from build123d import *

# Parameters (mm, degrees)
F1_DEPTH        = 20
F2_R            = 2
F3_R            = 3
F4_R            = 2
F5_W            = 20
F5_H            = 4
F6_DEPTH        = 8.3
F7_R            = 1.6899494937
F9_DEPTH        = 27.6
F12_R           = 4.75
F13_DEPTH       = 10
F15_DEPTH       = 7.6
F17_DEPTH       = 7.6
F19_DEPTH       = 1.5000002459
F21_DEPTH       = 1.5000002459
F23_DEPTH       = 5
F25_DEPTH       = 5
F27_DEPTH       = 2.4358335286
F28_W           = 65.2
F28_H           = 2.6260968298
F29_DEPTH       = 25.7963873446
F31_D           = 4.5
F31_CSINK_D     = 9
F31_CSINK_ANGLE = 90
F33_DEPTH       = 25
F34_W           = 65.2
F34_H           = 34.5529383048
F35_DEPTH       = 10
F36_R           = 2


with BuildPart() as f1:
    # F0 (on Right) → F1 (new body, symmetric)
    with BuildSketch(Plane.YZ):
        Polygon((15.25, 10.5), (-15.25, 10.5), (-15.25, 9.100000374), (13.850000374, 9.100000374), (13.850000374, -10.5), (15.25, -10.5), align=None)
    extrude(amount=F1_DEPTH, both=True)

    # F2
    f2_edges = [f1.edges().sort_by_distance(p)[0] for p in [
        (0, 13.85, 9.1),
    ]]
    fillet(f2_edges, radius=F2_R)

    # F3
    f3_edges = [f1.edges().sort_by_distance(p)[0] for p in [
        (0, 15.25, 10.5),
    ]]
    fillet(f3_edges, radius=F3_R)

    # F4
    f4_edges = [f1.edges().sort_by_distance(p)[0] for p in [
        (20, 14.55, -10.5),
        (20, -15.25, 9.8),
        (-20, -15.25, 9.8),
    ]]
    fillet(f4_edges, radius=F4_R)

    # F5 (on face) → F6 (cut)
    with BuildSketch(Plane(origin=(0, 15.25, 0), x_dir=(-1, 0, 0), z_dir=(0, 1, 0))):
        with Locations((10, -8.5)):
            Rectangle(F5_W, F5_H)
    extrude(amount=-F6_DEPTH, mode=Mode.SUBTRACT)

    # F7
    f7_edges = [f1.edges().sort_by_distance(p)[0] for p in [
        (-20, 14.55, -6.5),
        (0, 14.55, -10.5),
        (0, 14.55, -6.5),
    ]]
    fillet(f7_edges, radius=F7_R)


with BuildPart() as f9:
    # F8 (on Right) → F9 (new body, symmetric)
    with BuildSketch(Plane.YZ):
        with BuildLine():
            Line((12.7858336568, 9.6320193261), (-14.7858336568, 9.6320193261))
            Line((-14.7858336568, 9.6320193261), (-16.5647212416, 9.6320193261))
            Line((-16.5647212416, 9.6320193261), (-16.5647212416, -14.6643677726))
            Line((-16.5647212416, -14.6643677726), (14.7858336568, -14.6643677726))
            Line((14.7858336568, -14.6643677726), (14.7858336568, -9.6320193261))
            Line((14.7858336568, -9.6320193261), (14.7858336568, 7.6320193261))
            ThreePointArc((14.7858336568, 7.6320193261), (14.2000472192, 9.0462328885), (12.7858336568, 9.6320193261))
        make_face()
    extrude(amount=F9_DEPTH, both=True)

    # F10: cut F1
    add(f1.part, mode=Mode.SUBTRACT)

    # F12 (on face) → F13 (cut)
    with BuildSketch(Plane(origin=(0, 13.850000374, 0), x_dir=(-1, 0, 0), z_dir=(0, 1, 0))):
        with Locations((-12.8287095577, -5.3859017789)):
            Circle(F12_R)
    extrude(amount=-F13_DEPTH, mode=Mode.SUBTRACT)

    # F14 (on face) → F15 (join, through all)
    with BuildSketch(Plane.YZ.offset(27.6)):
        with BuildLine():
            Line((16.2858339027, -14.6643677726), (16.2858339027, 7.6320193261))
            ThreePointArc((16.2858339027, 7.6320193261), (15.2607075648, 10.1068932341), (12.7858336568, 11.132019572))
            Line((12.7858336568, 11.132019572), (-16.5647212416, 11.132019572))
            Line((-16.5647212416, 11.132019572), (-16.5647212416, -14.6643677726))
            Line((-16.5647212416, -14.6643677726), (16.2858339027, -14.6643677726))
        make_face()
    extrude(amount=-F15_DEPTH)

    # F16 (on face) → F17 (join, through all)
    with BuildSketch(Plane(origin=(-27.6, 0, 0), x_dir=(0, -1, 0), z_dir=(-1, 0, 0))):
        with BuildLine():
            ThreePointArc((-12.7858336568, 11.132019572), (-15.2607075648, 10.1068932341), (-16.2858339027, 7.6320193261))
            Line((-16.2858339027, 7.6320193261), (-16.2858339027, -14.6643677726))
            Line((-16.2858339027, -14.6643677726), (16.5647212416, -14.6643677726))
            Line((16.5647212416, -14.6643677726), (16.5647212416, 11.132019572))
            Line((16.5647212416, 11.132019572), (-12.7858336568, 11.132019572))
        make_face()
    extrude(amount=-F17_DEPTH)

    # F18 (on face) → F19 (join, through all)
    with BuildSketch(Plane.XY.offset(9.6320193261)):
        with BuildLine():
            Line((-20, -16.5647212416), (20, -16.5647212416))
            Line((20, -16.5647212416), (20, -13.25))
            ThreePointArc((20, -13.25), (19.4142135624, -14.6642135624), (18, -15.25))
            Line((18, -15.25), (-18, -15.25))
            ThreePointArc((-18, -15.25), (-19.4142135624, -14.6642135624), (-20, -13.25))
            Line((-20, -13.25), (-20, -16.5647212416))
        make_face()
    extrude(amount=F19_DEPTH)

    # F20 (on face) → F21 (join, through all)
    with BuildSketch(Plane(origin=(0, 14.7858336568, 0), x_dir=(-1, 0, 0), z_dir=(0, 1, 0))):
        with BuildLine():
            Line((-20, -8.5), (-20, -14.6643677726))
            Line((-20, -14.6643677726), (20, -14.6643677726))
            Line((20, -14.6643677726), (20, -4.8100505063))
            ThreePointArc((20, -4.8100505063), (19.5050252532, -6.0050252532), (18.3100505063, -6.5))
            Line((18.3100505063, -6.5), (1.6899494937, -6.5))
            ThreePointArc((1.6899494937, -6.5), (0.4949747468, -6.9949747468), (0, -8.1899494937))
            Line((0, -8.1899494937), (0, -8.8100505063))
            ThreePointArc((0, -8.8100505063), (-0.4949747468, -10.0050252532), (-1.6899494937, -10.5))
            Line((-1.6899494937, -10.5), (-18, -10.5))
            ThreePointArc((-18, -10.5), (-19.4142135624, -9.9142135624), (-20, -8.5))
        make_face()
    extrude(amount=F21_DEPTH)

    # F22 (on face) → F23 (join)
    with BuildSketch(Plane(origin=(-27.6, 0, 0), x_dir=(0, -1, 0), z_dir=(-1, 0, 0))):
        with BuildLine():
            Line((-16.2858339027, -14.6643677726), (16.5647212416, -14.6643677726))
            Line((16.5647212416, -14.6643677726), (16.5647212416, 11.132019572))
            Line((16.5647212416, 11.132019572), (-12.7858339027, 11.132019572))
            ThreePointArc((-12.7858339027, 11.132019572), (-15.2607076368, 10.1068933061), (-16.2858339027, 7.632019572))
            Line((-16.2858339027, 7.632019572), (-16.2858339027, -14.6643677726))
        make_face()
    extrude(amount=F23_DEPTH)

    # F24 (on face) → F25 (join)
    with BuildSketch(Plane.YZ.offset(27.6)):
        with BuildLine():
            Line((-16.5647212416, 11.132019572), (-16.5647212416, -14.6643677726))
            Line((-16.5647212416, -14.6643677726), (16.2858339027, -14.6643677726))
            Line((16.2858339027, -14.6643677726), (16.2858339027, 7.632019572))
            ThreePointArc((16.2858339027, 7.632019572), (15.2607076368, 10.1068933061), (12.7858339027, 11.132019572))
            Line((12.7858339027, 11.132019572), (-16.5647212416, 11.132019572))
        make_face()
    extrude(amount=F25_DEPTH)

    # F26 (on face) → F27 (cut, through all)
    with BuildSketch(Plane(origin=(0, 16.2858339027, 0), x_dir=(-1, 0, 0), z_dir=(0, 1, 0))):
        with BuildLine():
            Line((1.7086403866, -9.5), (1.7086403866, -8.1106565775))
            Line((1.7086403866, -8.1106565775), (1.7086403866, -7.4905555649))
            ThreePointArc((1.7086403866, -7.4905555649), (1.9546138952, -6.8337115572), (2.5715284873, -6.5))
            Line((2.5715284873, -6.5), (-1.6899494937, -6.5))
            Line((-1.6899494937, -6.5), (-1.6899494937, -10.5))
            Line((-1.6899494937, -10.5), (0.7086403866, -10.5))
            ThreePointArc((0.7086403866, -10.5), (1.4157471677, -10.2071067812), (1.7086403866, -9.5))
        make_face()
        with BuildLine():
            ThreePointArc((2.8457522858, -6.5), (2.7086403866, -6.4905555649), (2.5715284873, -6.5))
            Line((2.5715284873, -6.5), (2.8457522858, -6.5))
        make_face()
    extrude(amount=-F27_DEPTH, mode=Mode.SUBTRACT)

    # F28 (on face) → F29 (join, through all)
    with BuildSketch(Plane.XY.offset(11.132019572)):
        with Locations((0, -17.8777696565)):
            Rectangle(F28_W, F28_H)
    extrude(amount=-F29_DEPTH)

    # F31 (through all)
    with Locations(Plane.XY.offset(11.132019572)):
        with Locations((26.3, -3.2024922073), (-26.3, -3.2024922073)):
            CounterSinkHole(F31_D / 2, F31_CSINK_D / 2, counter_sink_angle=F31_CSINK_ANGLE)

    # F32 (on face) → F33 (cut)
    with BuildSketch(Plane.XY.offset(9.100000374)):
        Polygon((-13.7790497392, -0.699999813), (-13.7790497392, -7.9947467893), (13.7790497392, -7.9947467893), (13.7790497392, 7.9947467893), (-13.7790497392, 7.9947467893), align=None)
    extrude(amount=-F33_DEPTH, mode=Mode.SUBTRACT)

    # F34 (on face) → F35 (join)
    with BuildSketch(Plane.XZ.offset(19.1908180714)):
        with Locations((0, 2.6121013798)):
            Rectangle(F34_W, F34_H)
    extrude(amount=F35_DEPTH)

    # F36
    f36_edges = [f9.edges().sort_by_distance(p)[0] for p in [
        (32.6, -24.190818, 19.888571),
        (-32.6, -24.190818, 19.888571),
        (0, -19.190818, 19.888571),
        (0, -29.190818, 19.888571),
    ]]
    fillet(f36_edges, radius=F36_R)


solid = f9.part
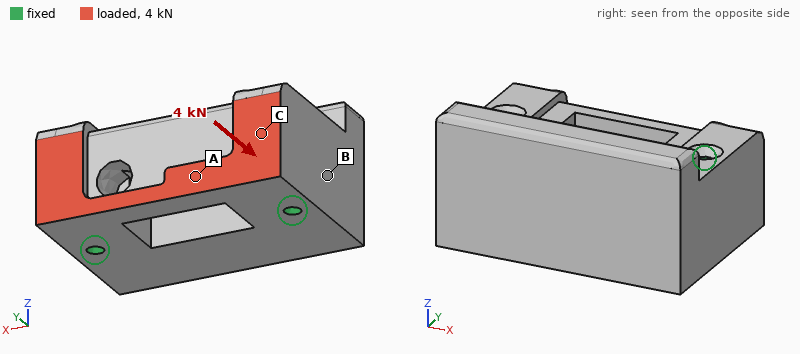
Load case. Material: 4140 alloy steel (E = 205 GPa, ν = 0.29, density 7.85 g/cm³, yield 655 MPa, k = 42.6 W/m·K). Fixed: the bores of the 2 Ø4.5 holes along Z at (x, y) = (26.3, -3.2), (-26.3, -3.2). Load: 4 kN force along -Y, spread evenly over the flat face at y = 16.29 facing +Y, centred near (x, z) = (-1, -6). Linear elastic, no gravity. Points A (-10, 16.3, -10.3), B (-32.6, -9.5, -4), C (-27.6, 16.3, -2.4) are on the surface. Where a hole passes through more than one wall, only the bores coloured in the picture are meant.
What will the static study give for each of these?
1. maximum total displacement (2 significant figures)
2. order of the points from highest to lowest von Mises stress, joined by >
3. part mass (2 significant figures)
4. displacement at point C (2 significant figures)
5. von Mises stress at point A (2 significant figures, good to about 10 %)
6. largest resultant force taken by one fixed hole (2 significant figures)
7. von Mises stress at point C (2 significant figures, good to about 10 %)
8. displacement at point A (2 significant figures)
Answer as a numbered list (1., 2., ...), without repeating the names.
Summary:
1. 3.8 µm
2. A > C > B
3. 520 g
4. 0.61 µm
5. 7.8 MPa
6. 2.1 kN
7. 5.4 MPa
8. 2.3 µm
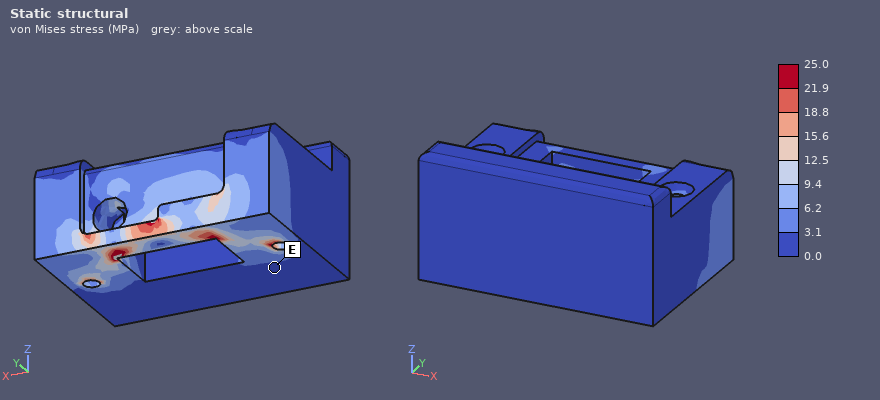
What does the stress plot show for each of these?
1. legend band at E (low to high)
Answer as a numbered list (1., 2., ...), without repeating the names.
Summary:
1. 0.0 to 3.1 MPa
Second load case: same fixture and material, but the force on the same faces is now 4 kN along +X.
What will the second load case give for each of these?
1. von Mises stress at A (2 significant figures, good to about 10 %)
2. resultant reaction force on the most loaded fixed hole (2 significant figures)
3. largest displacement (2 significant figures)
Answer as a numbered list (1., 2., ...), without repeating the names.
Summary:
1. 17 MPa
2. 2.3 kN
3. 4.5 µm
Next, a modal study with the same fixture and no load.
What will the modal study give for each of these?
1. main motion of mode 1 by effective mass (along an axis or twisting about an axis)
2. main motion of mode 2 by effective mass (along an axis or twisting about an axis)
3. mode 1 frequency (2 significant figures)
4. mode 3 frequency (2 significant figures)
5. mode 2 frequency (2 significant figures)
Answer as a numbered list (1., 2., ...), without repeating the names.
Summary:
1. along Z
2. along X
3. 11 kHz
4. 18 kHz
5. 16 kHz
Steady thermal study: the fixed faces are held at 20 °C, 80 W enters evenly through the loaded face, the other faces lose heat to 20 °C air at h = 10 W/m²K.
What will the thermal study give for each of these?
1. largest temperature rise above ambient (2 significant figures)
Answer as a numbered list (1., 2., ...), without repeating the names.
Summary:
1. 61 K
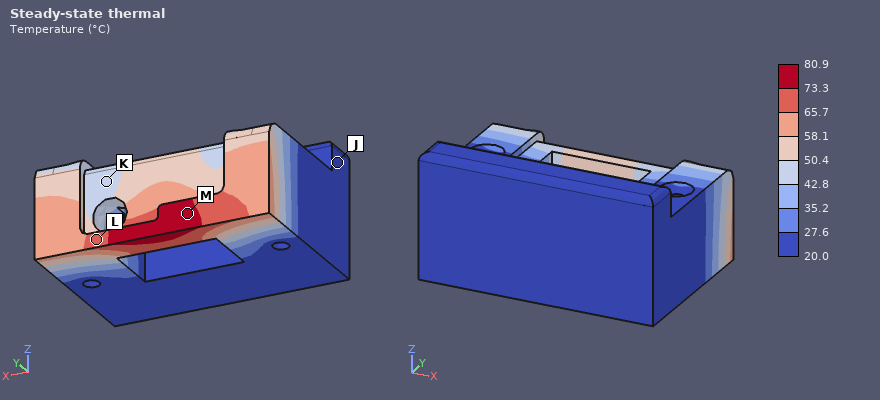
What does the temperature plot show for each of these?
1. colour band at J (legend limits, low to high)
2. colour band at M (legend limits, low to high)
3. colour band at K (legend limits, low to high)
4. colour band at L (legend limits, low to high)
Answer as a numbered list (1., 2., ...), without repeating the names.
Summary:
1. 20.0 to 27.6 °C
2. 73.3 to 80.9 °C
3. 42.8 to 50.4 °C
4. 65.7 to 73.3 °C
